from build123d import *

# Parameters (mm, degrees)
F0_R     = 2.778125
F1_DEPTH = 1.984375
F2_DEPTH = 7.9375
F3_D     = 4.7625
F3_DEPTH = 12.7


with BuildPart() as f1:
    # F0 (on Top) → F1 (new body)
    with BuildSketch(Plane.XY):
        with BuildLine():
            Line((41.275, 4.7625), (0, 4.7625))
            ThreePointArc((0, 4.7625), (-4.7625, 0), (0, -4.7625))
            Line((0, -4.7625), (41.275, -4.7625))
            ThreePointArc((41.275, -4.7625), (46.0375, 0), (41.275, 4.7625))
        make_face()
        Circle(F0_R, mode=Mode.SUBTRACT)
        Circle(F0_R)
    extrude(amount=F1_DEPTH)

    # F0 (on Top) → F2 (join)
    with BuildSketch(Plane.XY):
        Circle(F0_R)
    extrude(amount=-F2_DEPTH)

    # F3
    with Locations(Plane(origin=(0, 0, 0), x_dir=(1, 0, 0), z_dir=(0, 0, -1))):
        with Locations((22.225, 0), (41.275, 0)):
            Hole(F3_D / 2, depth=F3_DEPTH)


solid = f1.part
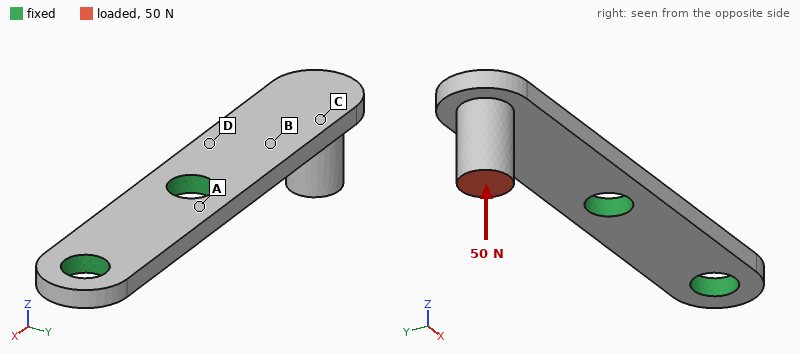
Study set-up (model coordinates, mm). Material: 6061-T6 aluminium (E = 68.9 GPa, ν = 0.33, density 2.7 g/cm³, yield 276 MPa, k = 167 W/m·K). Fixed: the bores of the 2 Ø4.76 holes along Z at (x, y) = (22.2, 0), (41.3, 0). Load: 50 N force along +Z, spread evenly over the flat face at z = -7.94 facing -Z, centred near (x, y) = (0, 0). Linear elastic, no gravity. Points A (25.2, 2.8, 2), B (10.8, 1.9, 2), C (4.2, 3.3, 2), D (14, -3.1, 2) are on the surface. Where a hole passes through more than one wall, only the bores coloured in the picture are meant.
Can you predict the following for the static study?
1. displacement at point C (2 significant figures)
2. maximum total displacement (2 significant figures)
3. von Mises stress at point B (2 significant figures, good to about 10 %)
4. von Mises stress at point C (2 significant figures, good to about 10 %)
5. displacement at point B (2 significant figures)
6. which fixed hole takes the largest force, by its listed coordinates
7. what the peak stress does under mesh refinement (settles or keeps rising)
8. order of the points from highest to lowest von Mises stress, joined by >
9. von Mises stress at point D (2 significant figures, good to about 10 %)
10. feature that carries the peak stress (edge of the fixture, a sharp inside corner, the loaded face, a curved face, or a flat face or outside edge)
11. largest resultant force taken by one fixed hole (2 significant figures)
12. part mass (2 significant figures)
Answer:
0.23 mm
0.45 mm
84 MPa
34 MPa
0.093 mm
(22.2, 0)
keeps rising
D > B > C > A
110 MPa
edge of the fixture
49 N
2.8 g
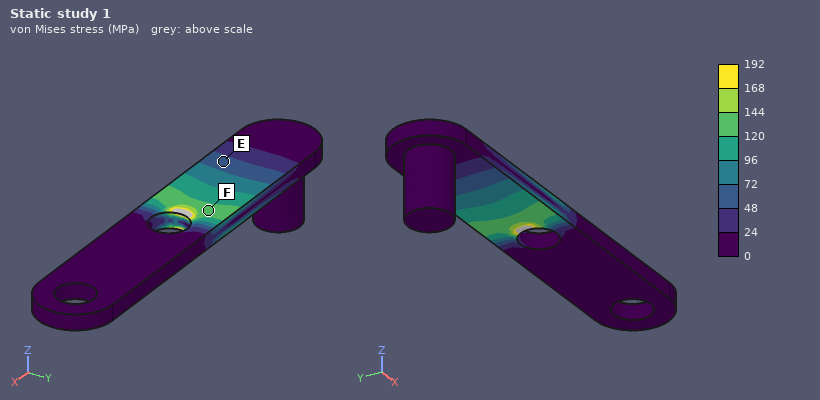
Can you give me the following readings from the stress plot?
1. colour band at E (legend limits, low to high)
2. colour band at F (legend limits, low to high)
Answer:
48 to 72 MPa
120 to 144 MPa
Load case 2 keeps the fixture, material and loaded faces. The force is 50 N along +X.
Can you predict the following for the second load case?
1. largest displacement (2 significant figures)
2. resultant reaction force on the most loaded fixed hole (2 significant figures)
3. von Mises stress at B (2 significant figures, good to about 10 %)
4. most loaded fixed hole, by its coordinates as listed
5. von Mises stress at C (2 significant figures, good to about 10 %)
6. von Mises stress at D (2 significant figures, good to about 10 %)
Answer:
0.32 mm
49 N
67 MPa
(22.2, 0)
66 MPa
68 MPa
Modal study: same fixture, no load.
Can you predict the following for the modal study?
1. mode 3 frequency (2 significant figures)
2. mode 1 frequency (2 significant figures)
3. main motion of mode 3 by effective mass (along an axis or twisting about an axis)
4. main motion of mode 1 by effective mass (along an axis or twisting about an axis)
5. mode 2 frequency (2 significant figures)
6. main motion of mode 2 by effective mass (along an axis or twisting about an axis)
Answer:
10 kHz
1900 Hz
along Y
along Z
5400 Hz
along Y
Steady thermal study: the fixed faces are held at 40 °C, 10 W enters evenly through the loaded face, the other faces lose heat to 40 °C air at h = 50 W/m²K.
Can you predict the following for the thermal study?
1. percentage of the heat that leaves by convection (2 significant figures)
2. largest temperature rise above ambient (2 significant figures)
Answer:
14 %
76 K
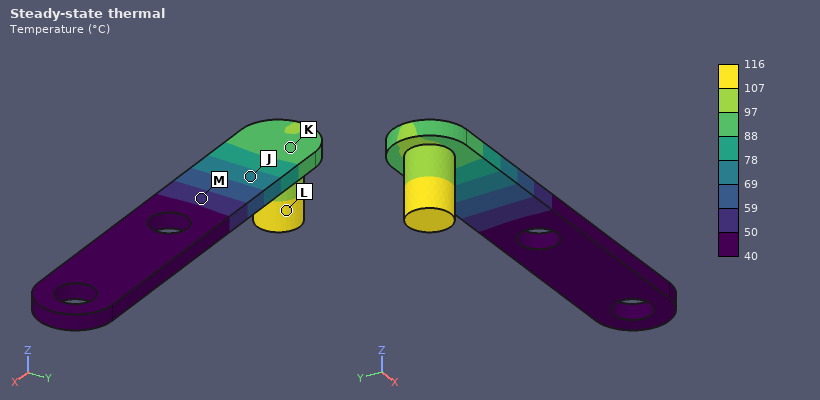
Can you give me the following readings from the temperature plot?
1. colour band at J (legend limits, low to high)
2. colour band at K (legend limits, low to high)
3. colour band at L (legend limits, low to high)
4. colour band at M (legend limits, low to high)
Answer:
69 to 78 °C
88 to 97 °C
107 to 116 °C
50 to 59 °C
